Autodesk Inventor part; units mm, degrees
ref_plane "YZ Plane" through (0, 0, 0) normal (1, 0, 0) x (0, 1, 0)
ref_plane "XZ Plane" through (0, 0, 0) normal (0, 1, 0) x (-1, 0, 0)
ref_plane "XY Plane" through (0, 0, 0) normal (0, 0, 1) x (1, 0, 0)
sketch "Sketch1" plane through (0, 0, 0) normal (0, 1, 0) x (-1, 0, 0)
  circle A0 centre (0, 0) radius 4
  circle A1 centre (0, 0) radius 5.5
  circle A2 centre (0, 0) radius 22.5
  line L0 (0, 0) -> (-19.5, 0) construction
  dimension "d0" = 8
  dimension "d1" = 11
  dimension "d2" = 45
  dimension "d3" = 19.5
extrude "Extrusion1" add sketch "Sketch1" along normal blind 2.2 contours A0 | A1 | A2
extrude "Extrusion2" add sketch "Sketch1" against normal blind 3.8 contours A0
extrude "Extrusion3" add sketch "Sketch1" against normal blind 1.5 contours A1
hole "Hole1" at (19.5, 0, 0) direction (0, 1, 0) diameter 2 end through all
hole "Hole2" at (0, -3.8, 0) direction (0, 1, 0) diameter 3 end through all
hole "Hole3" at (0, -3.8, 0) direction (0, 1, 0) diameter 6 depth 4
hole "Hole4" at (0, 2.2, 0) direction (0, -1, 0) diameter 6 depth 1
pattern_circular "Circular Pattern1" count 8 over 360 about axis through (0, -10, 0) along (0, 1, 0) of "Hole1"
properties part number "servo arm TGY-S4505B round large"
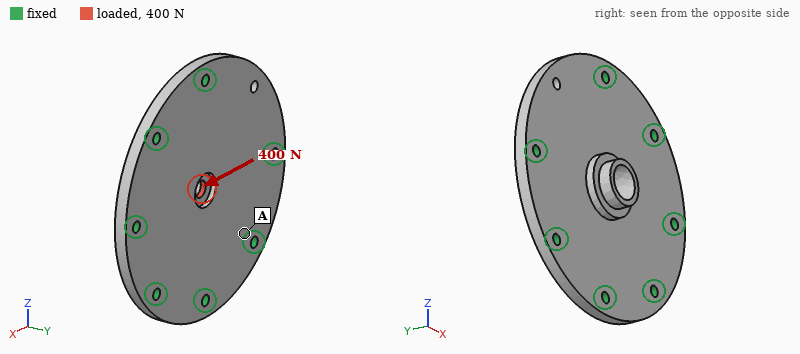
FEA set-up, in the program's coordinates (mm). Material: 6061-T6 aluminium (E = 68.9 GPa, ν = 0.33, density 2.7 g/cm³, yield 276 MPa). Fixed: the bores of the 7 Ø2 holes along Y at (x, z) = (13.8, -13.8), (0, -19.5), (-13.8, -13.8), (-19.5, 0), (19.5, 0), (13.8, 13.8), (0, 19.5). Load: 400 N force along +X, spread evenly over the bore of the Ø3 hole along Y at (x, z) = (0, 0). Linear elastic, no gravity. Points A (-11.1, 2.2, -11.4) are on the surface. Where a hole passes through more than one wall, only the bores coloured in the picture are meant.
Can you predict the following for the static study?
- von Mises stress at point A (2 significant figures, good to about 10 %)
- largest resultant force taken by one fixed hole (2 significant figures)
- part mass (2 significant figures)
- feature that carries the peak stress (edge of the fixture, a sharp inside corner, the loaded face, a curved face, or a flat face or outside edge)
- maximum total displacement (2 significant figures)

4.6 MPa
94 N
9.6 g
the loaded face
2.8 µm
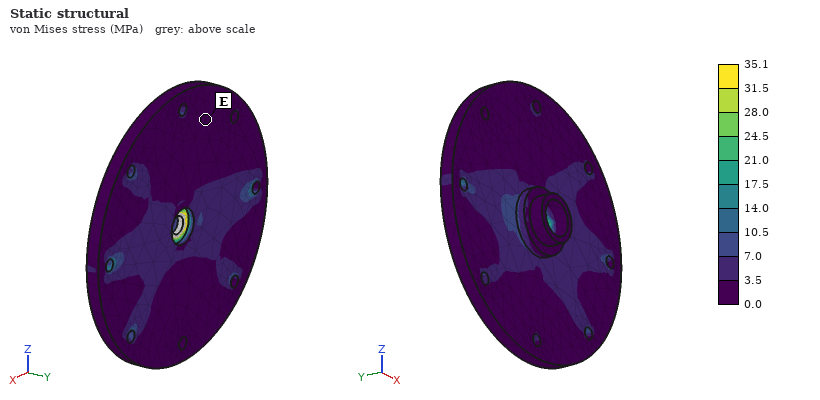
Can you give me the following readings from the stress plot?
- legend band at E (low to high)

0.0 to 3.5 MPa
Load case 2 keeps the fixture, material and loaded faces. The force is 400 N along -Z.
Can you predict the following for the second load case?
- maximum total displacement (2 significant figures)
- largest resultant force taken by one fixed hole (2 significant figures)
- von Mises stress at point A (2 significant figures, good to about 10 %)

2.8 µm
94 N
5.1 MPa
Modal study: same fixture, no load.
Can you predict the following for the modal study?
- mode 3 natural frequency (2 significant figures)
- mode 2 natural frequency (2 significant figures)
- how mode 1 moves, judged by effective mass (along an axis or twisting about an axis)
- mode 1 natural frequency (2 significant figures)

24 kHz
13 kHz
along Y
11 kHz
